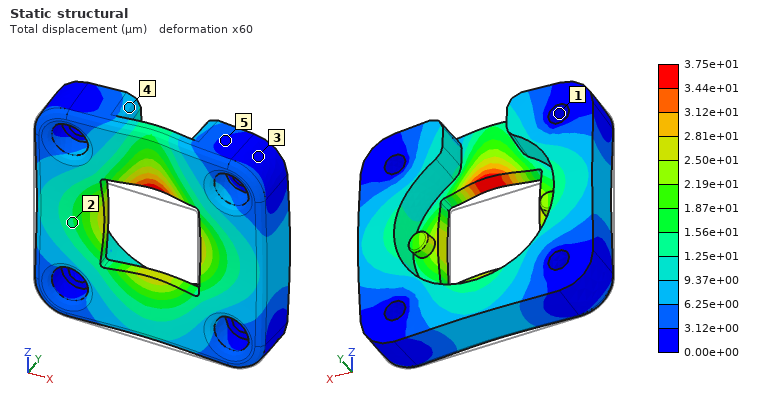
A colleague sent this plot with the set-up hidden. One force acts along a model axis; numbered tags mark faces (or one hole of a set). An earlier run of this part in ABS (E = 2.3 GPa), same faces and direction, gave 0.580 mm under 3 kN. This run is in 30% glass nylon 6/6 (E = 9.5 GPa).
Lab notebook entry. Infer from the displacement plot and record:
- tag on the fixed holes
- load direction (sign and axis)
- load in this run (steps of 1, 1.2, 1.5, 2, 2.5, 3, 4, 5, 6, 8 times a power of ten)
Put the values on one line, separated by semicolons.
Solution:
1; +Y; 800 N
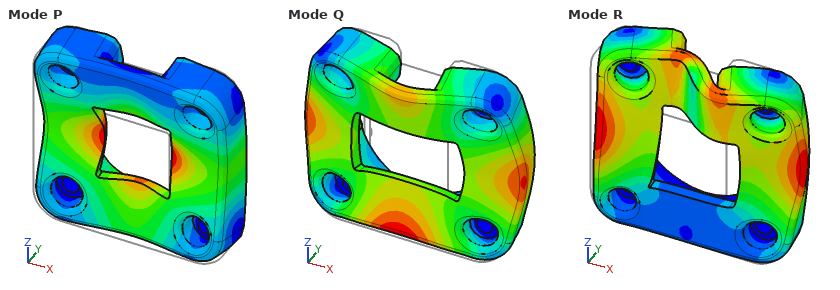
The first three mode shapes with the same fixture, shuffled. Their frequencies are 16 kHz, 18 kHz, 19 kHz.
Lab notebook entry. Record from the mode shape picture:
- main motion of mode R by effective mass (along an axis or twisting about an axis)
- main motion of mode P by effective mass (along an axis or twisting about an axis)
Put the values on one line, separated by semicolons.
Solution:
along X; along Y
